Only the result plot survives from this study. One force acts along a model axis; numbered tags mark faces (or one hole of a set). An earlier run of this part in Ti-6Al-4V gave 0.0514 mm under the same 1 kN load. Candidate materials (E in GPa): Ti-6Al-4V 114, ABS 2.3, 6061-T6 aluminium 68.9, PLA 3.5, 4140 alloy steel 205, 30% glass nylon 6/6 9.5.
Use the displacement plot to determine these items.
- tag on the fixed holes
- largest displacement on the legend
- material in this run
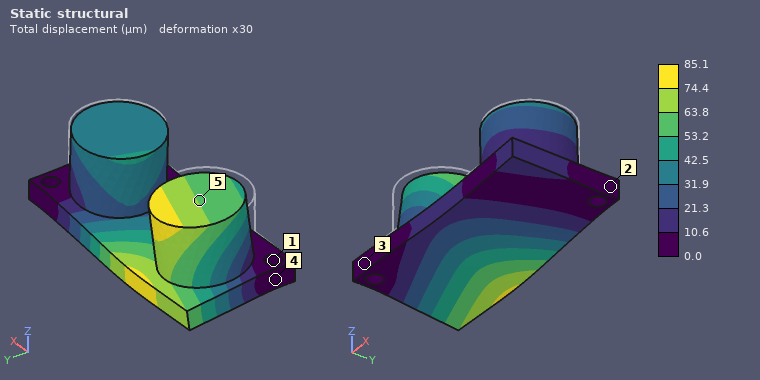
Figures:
1
85.1 µm
6061-T6 aluminium
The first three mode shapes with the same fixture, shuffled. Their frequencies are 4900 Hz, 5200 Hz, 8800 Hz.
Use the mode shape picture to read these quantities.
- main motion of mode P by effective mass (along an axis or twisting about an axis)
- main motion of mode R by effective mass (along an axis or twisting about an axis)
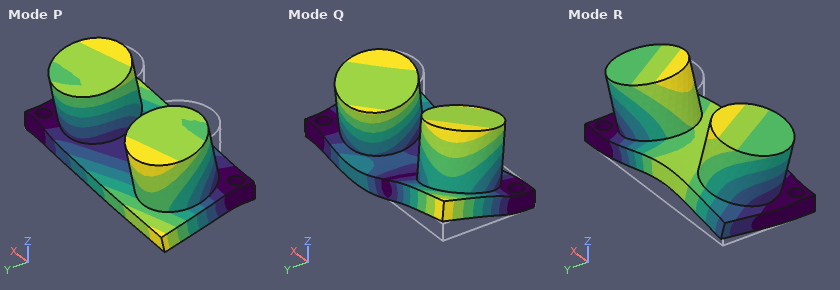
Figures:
along Y
along Z
